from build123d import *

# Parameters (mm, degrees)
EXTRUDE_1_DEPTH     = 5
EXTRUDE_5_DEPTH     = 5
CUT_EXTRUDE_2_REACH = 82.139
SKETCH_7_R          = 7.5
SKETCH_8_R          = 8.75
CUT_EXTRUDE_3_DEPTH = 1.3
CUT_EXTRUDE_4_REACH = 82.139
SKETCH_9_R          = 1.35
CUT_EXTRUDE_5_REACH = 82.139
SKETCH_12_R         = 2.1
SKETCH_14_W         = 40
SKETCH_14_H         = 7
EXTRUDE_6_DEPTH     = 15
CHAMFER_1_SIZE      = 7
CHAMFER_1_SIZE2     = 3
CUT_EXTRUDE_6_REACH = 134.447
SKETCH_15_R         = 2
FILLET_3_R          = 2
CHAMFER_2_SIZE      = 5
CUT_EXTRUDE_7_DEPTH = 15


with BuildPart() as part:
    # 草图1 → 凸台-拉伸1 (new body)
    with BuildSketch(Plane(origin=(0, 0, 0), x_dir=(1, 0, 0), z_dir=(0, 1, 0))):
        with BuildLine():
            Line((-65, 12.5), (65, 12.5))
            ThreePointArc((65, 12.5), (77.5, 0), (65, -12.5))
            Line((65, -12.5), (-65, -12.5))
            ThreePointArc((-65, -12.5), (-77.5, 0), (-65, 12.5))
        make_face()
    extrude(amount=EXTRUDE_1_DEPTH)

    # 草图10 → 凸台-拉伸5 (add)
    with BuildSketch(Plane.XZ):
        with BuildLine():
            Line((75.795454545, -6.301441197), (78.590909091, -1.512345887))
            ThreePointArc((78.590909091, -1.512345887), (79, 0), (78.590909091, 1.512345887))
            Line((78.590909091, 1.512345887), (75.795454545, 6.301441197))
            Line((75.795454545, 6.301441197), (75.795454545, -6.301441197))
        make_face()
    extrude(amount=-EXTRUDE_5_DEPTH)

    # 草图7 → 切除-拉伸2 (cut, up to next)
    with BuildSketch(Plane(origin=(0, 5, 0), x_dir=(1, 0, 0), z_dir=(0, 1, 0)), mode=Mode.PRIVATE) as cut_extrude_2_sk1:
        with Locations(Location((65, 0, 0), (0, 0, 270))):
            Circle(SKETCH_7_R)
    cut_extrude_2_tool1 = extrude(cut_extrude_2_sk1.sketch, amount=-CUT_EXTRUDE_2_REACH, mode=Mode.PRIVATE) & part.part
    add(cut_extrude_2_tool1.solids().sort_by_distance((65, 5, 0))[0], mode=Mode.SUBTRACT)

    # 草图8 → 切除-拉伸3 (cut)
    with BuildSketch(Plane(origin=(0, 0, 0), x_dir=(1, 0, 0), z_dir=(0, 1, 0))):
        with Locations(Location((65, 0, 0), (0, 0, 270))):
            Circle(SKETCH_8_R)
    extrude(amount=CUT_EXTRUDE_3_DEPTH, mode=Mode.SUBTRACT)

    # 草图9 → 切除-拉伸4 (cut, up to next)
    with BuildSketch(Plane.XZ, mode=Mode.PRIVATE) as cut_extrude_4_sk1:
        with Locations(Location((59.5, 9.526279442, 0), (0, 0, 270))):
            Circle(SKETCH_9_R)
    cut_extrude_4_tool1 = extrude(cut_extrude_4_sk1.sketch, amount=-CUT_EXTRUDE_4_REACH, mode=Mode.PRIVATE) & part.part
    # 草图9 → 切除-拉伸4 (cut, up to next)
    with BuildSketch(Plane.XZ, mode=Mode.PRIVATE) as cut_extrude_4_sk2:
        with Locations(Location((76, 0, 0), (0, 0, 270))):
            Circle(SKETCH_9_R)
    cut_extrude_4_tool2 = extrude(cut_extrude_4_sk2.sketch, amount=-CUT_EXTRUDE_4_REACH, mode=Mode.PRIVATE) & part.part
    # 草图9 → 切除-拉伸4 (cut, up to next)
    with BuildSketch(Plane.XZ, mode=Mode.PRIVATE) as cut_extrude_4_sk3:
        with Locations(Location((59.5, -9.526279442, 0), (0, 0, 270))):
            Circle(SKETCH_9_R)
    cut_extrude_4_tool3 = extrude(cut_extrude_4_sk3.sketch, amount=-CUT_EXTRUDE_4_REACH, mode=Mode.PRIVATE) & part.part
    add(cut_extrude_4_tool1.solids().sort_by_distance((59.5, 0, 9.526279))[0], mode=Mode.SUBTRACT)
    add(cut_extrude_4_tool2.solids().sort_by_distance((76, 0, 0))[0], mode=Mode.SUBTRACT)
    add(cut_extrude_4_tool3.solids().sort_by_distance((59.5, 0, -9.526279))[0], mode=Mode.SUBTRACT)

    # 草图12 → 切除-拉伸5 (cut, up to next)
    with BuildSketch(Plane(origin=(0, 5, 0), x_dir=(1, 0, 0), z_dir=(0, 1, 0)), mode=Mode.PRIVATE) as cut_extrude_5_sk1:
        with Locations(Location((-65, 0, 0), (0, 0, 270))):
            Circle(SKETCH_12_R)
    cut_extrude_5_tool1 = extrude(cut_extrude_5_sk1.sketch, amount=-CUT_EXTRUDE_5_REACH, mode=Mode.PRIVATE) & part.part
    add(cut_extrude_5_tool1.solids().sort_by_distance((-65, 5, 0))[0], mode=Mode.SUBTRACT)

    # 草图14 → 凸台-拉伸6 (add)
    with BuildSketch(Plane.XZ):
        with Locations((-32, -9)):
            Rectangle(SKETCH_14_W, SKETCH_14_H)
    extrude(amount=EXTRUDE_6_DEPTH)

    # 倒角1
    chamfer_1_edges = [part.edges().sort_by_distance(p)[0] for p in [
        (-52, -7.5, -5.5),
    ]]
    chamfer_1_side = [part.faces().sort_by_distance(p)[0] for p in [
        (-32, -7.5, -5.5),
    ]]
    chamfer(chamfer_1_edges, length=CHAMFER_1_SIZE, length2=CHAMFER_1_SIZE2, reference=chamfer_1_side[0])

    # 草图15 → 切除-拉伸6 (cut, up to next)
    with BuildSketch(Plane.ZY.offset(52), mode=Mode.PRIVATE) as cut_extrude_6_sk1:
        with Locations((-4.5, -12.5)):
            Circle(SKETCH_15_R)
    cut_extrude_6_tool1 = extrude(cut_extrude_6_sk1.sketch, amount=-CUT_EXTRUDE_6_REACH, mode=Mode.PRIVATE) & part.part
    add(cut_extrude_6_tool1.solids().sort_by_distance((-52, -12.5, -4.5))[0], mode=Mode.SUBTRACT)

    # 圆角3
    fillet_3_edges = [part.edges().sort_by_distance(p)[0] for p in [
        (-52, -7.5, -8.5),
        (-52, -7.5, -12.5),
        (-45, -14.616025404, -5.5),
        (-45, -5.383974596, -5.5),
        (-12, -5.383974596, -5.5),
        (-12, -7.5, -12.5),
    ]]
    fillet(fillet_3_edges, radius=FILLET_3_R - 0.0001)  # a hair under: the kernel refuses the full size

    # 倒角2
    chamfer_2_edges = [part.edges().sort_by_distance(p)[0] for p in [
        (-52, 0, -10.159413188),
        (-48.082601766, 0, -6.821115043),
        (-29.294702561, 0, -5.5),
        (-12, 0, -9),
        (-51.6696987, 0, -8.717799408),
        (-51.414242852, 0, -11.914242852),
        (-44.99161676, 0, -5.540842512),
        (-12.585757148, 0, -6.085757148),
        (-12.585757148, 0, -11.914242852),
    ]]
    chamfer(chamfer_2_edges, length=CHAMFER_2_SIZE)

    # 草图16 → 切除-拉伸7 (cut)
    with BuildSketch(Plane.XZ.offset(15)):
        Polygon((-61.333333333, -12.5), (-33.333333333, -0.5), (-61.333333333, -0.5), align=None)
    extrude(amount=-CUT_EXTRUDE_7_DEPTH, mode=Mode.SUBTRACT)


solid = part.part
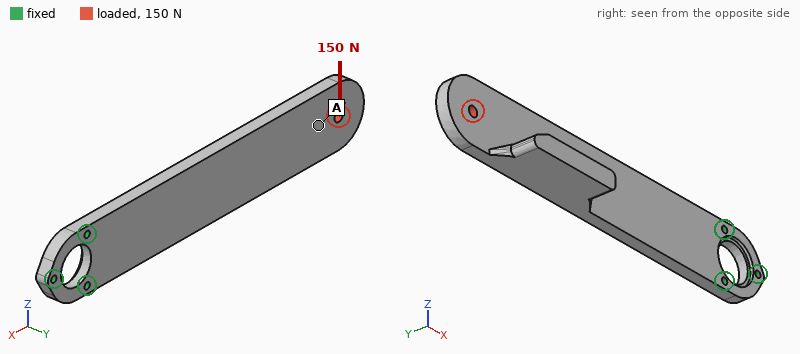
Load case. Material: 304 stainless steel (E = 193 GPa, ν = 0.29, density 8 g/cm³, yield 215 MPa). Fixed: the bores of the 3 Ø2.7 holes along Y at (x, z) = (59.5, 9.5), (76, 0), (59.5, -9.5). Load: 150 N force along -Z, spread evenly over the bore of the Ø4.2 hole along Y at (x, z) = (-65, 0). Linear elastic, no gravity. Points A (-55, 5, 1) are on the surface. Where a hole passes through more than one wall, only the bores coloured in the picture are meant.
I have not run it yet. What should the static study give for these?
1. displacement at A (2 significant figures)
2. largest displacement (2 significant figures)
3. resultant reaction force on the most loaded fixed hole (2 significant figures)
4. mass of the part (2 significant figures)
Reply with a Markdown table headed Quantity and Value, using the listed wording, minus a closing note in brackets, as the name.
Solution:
| Quantity | Value |
|---|---|
| displacement at A | 69 µm |
| largest displacement | 90 µm |
| resultant reaction force on the most loaded fixed hole | 960 N |
| mass of the part | 180 g |
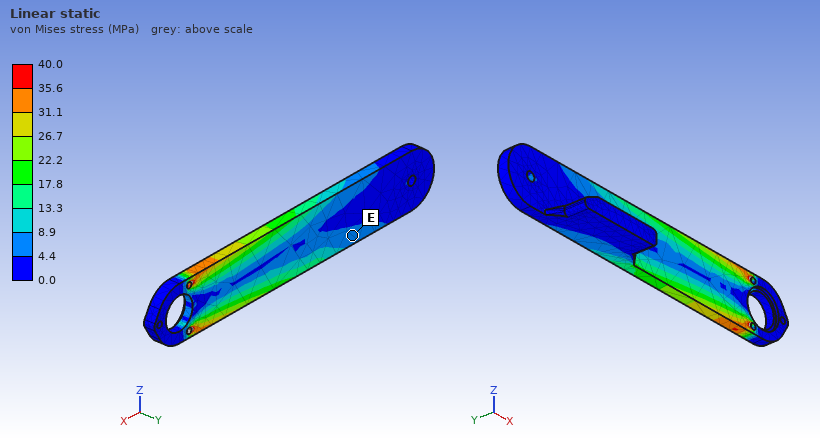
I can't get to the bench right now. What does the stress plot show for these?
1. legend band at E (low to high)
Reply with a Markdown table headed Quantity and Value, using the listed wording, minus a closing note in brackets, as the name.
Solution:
| Quantity | Value |
|---|---|
| legend band at E | 4.4 to 8.9 MPa |
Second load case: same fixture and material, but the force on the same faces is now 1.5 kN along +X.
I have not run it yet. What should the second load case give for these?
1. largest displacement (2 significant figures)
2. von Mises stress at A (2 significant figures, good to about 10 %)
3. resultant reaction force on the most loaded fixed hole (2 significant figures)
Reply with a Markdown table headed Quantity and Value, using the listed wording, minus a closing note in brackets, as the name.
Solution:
| Quantity | Value |
|---|---|
| largest displacement | 12 µm |
| von Mises stress at A | 17 MPa |
| resultant reaction force on the most loaded fixed hole | 780 N |
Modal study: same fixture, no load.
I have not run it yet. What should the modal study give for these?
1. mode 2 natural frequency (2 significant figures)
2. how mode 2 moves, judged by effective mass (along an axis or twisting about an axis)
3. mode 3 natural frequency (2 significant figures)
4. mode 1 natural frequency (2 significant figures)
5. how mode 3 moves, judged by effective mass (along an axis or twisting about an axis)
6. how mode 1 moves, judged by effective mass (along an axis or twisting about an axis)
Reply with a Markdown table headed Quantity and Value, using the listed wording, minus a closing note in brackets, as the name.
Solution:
| Quantity | Value |
|---|---|
| mode 2 natural frequency | 910 Hz |
| how mode 2 moves, judged by effective mass | along Z |
| mode 3 natural frequency | 1400 Hz |
| mode 1 natural frequency | 180 Hz |
| how mode 3 moves, judged by effective mass | along Y |
| how mode 1 moves, judged by effective mass | along Y |
